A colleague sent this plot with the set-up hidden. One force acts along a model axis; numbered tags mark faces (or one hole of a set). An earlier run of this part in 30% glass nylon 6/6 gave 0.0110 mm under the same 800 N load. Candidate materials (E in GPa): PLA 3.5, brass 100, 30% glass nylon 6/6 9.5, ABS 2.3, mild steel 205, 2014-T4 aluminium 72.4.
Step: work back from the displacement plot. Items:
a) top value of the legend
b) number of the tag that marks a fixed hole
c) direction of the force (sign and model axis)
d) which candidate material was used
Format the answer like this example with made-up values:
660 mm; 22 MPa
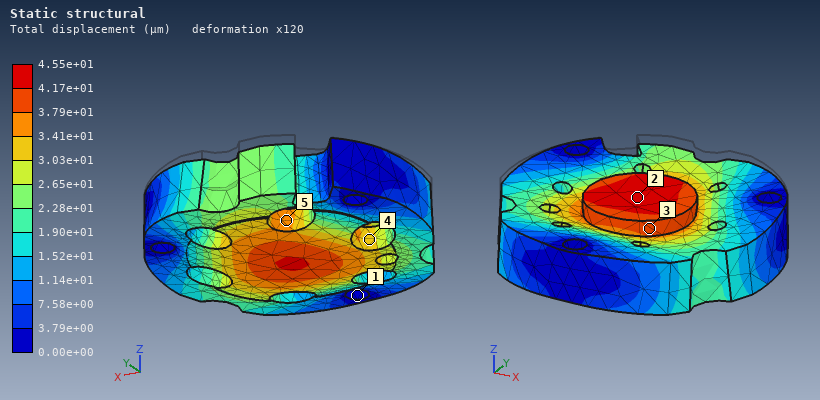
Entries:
4.55e+01 µm; 1; -Z; ABS
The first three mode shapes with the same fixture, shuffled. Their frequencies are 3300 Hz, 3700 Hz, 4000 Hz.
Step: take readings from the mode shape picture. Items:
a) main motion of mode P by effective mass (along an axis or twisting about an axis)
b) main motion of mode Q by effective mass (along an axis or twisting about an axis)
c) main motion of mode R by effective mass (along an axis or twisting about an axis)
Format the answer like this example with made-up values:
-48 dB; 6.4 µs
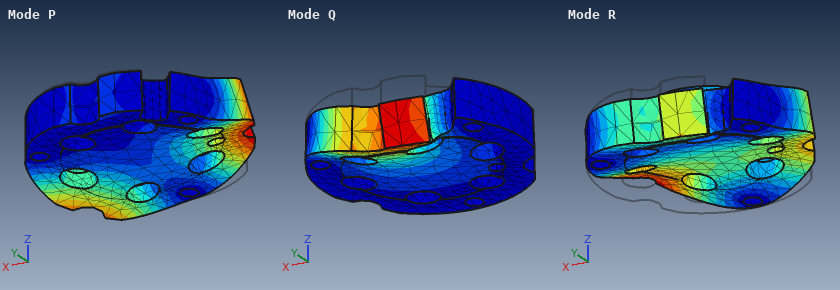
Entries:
twisting about Y; along Z; along Z
